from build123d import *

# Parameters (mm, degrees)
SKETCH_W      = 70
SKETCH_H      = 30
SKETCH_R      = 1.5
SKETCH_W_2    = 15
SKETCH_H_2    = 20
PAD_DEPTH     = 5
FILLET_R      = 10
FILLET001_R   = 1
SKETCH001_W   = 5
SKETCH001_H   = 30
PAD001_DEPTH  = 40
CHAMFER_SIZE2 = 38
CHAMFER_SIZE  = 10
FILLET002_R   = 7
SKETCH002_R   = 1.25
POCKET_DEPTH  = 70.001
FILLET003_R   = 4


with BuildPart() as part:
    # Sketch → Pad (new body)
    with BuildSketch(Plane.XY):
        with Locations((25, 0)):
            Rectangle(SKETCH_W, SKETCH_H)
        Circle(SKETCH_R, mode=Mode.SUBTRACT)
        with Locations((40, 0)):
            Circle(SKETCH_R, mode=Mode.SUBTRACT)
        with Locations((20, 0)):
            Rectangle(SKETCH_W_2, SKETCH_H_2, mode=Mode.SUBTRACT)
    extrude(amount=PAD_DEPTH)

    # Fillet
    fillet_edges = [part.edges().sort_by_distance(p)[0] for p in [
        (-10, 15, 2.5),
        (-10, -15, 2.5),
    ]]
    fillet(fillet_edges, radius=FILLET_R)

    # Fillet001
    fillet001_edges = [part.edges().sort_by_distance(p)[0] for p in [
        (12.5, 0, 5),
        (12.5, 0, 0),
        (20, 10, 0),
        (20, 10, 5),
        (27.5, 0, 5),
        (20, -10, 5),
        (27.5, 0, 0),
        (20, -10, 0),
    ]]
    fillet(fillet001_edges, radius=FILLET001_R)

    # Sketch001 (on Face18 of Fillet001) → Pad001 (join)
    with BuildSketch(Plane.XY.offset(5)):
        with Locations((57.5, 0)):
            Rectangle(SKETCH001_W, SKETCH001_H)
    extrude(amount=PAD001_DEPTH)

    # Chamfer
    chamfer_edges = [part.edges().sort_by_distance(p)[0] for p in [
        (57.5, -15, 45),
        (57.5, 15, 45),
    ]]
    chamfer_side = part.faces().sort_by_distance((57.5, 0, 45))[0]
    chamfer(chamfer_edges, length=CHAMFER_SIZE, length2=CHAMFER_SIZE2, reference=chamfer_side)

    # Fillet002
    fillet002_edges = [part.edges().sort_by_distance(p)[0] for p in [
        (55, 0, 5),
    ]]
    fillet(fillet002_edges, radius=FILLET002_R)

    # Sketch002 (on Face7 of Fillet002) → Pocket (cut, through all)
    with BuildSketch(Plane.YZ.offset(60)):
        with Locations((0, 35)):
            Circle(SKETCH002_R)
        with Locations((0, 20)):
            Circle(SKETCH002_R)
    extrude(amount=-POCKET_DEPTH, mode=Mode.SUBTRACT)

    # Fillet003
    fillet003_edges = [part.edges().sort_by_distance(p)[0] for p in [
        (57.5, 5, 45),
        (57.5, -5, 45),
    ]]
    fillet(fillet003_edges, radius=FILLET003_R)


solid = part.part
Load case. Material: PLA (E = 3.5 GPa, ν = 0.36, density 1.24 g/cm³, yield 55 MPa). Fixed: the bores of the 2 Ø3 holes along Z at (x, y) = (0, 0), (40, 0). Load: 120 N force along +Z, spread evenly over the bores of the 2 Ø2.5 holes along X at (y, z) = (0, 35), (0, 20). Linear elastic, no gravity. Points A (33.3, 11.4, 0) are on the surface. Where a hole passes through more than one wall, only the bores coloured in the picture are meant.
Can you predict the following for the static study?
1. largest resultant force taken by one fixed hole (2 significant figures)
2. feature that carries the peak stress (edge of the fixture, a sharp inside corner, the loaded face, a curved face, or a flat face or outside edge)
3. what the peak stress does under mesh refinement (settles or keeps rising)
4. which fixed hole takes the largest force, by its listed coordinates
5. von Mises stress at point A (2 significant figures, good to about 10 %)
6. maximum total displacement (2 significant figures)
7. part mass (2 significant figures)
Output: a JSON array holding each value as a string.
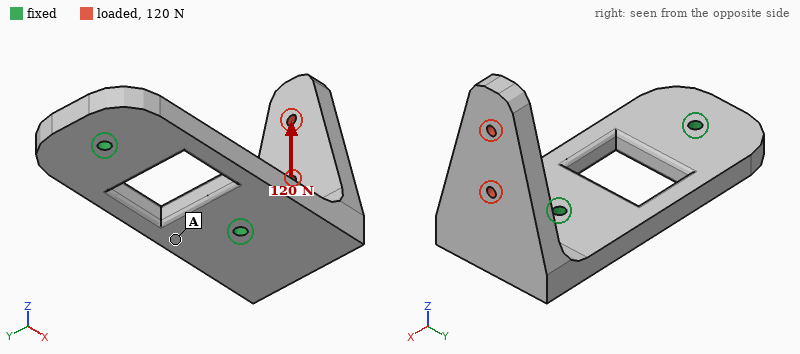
["130 N", "edge of the fixture", "keeps rising", "(40, 0)", "4.1 MPa", "0.92 mm", "16 g"]
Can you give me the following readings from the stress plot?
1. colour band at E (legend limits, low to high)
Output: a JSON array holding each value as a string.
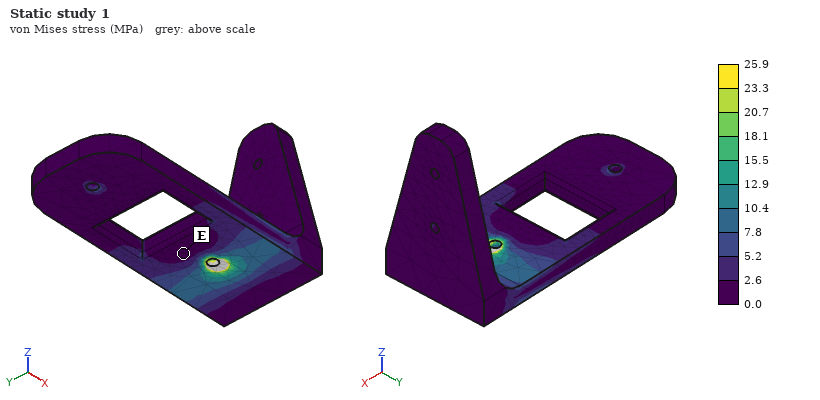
["0.0 to 2.6 MPa"]
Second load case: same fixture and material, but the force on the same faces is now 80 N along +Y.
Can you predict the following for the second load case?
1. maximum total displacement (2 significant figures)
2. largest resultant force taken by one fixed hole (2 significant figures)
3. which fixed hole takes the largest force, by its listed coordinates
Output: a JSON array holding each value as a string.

["0.89 mm", "100 N", "(40, 0)"]
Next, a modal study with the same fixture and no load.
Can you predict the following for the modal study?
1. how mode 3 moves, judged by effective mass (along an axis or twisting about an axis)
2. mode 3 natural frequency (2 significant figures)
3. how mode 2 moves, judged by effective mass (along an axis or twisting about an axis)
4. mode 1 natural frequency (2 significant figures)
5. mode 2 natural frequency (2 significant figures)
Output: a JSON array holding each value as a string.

["along Z", "2000 Hz", "along Y", "660 Hz", "920 Hz"]
